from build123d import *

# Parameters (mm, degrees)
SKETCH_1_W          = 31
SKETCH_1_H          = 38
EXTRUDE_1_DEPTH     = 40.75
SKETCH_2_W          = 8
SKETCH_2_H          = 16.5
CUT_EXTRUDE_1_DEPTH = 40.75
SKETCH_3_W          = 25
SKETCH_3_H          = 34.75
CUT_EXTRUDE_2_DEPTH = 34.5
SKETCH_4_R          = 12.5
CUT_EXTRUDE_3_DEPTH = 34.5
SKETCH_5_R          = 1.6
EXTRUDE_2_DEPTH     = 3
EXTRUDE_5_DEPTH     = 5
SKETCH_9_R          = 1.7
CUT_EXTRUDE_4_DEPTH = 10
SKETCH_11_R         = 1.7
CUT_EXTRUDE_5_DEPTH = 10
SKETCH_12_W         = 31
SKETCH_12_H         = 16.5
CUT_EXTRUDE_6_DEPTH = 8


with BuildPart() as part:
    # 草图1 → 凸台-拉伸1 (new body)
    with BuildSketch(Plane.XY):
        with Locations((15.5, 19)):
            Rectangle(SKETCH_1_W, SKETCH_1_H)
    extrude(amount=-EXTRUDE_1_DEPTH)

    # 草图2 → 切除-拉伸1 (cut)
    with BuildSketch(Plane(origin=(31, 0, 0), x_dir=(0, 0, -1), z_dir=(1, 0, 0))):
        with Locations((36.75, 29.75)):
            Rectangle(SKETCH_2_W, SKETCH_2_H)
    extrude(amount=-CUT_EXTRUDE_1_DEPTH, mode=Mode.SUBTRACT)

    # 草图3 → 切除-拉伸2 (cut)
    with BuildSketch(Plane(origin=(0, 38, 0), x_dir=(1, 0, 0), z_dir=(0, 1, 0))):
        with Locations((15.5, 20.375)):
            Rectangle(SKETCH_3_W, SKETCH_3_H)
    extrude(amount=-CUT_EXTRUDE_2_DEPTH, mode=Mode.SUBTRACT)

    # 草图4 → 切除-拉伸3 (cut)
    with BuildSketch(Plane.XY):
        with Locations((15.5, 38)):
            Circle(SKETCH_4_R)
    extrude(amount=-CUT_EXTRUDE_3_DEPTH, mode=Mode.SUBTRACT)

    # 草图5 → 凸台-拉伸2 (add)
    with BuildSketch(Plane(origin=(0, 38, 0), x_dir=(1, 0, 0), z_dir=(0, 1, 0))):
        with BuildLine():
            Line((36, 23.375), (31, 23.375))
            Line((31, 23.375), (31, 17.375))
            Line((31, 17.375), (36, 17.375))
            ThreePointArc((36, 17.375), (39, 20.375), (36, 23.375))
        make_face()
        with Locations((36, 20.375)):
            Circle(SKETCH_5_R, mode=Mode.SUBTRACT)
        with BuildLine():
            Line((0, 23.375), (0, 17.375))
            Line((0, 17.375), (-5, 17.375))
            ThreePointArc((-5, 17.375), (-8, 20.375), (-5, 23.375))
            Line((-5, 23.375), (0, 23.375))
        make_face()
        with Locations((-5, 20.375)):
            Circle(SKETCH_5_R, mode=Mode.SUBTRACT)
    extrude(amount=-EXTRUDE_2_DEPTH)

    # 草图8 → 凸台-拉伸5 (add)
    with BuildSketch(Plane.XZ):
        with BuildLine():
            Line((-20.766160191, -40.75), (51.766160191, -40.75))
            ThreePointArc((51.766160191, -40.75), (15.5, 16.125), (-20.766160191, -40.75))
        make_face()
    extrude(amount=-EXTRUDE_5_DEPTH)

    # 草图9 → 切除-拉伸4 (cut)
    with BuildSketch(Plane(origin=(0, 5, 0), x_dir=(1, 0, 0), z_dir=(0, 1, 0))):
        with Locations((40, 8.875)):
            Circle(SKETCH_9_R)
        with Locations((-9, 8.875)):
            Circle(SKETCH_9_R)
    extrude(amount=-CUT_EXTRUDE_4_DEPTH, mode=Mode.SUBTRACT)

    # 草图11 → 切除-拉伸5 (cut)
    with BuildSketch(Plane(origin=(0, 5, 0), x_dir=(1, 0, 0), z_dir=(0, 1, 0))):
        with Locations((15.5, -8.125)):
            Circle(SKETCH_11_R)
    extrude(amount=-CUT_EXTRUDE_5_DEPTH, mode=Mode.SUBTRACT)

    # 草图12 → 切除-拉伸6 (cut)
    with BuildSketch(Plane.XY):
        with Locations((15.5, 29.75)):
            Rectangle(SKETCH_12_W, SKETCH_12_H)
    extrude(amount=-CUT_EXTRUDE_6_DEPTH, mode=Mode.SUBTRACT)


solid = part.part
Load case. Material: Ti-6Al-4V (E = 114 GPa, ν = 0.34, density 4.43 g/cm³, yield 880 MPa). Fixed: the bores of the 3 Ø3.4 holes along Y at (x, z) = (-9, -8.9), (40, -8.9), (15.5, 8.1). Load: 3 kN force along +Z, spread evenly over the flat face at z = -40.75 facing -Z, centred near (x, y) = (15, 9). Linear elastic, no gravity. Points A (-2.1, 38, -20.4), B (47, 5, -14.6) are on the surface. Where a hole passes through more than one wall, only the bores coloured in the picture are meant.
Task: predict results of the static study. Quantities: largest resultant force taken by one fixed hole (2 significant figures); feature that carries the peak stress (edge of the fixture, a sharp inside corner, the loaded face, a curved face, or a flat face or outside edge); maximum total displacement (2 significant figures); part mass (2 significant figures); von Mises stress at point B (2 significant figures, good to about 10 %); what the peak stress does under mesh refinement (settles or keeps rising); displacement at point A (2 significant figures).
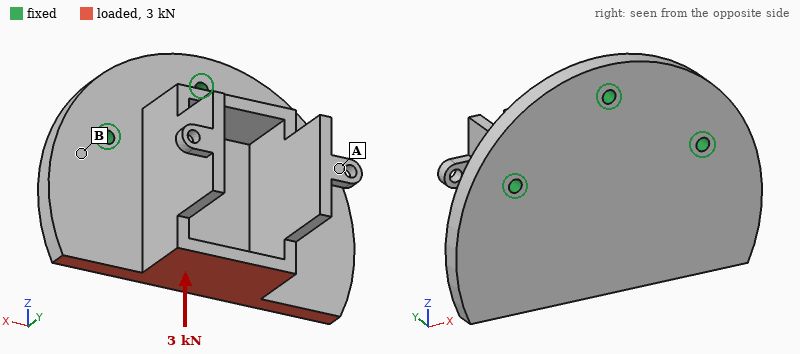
1.1 kN
edge of the fixture
71 µm
120 g
19 MPa
keeps rising
47 µm
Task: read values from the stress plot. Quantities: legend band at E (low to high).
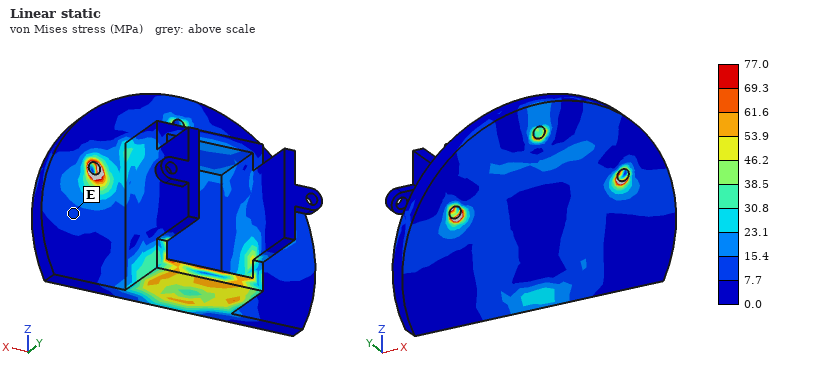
7.7 to 15.4 MPa
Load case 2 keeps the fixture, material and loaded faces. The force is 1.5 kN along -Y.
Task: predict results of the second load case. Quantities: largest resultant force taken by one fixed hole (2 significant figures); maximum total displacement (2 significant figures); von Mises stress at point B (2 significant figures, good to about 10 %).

1.4 kN
0.13 mm
51 MPa
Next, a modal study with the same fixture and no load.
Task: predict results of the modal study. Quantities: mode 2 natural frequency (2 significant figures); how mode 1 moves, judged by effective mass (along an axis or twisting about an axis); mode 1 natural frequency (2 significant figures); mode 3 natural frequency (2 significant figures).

3200 Hz
along Y
2900 Hz
3400 Hz
